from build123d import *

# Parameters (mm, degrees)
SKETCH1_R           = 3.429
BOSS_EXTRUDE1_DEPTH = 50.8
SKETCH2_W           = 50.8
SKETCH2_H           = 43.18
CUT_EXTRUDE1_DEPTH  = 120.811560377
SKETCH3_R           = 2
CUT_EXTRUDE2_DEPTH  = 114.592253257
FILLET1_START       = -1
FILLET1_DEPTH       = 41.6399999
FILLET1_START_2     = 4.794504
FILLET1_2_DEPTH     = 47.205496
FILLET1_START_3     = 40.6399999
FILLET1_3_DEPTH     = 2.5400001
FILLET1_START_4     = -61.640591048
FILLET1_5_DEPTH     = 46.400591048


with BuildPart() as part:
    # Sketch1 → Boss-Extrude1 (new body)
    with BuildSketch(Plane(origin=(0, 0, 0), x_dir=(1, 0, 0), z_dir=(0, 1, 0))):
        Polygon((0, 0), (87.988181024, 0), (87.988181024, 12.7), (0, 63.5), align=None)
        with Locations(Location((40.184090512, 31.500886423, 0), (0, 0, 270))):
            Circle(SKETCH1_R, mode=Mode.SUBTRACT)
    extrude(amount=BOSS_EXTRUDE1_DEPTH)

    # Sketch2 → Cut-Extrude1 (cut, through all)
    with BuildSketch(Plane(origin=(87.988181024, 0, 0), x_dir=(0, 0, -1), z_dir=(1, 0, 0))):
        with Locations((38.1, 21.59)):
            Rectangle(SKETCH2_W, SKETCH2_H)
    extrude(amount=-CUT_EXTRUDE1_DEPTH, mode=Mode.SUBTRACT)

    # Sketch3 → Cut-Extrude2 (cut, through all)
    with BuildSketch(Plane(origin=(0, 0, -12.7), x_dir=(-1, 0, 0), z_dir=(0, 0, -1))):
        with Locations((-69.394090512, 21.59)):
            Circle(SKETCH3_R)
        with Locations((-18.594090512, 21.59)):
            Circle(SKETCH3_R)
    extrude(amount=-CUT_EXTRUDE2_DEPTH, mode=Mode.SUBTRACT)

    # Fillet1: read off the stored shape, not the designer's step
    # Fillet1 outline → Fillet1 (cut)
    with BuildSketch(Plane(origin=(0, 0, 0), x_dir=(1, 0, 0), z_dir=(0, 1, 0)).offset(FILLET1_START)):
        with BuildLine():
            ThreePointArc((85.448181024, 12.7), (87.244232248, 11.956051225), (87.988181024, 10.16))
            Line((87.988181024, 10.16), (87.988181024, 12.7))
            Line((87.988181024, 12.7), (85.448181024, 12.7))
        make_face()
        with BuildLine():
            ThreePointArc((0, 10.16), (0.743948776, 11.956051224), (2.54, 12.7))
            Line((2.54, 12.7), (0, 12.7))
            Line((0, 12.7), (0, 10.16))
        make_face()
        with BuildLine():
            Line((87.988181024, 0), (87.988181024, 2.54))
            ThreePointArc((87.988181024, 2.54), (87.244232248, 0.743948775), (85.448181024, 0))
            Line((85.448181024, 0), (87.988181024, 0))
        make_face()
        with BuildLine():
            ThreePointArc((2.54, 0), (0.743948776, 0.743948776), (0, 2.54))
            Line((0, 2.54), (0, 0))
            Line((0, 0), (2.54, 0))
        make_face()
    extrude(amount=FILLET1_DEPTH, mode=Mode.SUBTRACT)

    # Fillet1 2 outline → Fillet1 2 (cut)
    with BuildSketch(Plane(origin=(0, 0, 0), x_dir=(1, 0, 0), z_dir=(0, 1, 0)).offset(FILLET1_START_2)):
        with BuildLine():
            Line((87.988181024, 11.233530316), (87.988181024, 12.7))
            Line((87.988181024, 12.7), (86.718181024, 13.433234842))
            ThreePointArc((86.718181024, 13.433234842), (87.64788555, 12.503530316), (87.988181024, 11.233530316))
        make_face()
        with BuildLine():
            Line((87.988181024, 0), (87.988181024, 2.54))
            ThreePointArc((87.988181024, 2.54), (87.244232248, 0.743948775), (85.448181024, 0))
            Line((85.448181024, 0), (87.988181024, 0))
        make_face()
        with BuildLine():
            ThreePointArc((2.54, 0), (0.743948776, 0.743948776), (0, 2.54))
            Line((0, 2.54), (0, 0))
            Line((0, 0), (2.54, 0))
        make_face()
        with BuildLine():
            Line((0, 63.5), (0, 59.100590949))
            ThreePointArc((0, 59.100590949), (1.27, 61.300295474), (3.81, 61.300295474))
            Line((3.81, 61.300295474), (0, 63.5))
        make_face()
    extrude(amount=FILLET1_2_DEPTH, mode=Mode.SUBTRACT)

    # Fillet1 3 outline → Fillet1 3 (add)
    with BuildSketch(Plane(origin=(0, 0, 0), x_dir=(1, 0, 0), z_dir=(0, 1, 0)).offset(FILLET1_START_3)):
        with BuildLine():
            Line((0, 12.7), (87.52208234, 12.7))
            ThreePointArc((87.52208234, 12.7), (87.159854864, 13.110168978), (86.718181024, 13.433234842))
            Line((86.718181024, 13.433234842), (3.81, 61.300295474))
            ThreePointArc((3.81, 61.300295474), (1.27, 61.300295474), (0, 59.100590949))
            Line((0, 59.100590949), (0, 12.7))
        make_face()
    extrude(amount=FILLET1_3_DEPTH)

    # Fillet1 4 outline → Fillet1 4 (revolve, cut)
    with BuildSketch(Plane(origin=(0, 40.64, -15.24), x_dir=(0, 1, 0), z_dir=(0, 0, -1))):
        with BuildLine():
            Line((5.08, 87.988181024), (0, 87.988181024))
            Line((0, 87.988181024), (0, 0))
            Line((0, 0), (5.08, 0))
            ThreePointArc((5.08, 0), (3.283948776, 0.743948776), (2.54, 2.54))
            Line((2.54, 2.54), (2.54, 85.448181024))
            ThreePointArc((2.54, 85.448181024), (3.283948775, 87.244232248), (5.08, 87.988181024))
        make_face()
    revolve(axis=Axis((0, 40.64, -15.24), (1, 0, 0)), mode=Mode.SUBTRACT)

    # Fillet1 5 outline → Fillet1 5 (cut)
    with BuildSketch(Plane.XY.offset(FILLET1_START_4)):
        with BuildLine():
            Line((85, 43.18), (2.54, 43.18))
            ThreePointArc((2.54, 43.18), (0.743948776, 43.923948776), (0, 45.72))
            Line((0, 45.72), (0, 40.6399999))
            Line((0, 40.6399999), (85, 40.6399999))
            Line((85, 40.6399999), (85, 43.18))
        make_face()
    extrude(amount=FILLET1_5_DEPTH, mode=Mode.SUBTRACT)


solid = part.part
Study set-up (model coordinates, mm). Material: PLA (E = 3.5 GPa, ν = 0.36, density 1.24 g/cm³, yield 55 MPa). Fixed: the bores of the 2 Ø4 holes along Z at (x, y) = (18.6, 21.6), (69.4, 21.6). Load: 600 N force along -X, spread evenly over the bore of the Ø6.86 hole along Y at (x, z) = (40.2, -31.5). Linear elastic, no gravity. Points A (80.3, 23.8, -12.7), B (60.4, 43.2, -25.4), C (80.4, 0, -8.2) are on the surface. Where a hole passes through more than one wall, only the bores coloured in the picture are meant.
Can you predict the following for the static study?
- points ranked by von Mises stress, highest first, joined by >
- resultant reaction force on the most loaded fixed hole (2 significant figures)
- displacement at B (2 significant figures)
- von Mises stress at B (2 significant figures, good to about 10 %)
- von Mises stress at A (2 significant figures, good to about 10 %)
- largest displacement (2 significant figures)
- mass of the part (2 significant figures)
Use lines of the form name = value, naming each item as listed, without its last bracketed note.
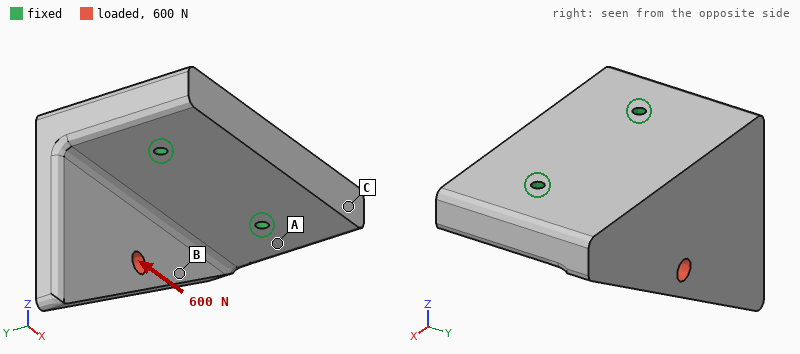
points ranked by von Mises stress, highest first, joined by > = B > A > C
resultant reaction force on the most loaded fixed hole = 490 N
displacement at B = 0.091 mm
von Mises stress at B = 4.6 MPa
von Mises stress at A = 2.1 MPa
largest displacement = 0.25 mm
mass of the part = 90 g
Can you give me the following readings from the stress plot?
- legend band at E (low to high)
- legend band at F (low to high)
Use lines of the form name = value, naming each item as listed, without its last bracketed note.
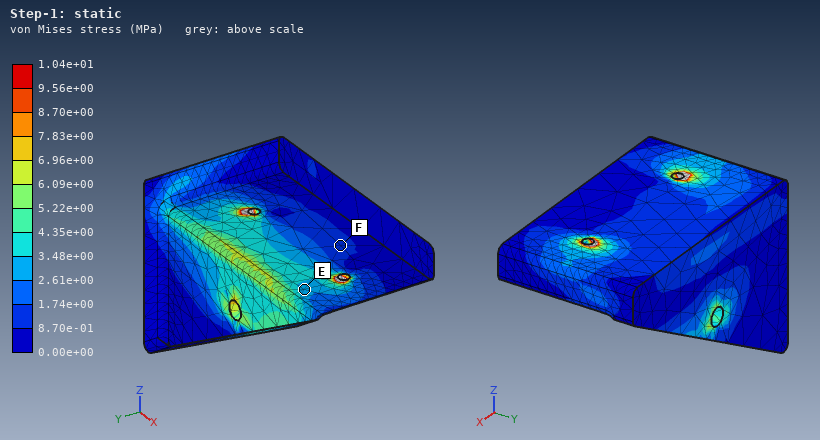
legend band at E = 2.61e+00 to 3.48e+00 MPa
legend band at F = 8.70e-01 to 1.74e+00 MPa
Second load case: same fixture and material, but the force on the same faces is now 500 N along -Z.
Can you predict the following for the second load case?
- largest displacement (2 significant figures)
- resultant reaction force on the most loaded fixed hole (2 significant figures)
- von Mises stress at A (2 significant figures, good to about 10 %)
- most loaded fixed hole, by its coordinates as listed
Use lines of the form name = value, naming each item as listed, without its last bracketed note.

largest displacement = 0.34 mm
resultant reaction force on the most loaded fixed hole = 280 N
von Mises stress at A = 2.2 MPa
most loaded fixed hole, by its coordinates as listed = (18.6, 21.6)
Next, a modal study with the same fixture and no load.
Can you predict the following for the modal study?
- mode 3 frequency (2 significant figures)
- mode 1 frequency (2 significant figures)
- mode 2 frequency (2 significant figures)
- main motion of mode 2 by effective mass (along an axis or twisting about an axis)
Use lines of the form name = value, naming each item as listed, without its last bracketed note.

mode 3 frequency = 1900 Hz
mode 1 frequency = 900 Hz
mode 2 frequency = 1800 Hz
main motion of mode 2 by effective mass = along Z
